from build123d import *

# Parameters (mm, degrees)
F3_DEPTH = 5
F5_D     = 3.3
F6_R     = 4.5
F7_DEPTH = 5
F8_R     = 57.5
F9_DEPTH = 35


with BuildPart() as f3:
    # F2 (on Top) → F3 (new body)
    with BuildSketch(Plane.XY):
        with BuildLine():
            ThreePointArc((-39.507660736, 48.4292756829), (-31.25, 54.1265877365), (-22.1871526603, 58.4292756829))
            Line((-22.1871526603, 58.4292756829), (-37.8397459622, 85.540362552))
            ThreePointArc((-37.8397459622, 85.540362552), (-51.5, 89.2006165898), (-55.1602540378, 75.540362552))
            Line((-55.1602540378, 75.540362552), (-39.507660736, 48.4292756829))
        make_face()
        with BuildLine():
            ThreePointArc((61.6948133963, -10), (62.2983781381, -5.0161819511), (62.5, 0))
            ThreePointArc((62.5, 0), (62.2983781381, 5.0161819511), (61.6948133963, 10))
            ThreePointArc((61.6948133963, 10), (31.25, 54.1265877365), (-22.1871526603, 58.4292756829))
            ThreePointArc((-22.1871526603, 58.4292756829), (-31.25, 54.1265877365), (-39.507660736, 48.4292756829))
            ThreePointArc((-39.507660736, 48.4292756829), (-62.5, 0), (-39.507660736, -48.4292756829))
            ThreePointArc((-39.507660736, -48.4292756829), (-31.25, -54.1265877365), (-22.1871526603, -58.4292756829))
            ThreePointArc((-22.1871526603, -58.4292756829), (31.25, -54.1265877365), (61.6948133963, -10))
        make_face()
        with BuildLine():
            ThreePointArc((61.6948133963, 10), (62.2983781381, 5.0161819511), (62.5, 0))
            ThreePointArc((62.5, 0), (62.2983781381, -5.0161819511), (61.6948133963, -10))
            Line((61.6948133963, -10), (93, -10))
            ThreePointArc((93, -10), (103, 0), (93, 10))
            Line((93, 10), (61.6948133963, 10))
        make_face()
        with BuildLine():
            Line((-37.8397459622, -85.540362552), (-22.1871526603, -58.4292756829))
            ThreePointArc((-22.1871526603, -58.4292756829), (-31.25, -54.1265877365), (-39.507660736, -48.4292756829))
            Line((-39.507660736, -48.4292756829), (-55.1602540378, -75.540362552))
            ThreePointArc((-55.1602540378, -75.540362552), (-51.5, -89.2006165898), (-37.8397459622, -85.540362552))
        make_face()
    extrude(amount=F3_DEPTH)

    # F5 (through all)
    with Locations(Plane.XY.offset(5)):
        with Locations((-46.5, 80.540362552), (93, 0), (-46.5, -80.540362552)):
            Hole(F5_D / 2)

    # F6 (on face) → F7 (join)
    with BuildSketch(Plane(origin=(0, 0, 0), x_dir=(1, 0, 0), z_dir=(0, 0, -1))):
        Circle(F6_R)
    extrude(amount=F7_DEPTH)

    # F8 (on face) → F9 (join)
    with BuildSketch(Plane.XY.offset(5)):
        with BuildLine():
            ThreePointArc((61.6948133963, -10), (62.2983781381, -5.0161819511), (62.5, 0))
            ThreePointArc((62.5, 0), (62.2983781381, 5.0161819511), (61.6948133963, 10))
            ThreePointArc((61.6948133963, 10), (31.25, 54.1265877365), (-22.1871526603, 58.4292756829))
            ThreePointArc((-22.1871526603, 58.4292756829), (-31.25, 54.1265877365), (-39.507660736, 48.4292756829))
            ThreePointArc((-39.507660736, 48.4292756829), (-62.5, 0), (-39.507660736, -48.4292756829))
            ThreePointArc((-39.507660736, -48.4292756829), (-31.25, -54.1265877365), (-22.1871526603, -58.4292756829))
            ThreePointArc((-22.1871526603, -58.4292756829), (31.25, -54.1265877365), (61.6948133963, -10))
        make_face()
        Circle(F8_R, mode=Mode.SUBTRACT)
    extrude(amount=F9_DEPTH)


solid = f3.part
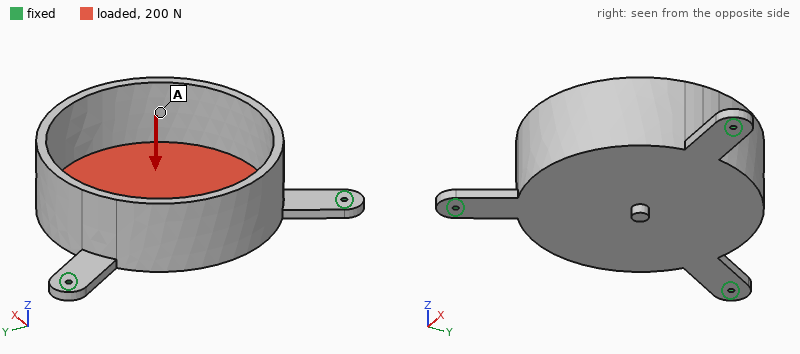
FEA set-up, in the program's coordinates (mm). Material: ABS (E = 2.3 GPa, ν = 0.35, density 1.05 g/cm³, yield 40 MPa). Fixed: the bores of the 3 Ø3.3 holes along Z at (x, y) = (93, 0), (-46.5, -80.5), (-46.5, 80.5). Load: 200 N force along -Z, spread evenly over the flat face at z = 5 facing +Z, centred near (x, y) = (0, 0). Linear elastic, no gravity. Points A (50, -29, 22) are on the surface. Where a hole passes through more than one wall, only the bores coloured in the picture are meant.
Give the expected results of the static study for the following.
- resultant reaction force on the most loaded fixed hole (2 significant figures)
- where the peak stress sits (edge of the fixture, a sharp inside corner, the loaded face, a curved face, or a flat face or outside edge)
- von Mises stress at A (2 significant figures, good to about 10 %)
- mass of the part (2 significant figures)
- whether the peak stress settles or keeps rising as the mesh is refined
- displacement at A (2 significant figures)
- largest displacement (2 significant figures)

72 N
edge of the fixture
1.1 MPa
150 g
keeps rising
0.61 mm
0.83 mm
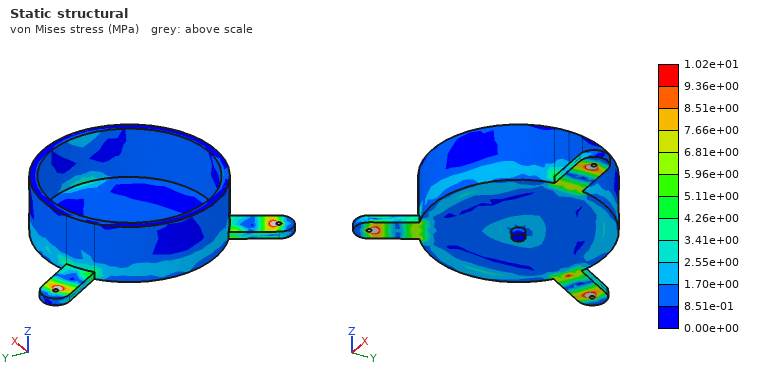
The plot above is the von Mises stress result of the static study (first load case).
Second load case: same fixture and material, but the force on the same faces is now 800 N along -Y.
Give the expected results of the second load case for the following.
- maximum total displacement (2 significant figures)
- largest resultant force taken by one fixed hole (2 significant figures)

0.32 mm
410 N
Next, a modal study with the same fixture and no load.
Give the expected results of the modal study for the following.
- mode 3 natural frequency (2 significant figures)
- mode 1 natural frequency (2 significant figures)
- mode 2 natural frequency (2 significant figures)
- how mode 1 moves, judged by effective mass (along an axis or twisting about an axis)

290 Hz
250 Hz
290 Hz
along Z
